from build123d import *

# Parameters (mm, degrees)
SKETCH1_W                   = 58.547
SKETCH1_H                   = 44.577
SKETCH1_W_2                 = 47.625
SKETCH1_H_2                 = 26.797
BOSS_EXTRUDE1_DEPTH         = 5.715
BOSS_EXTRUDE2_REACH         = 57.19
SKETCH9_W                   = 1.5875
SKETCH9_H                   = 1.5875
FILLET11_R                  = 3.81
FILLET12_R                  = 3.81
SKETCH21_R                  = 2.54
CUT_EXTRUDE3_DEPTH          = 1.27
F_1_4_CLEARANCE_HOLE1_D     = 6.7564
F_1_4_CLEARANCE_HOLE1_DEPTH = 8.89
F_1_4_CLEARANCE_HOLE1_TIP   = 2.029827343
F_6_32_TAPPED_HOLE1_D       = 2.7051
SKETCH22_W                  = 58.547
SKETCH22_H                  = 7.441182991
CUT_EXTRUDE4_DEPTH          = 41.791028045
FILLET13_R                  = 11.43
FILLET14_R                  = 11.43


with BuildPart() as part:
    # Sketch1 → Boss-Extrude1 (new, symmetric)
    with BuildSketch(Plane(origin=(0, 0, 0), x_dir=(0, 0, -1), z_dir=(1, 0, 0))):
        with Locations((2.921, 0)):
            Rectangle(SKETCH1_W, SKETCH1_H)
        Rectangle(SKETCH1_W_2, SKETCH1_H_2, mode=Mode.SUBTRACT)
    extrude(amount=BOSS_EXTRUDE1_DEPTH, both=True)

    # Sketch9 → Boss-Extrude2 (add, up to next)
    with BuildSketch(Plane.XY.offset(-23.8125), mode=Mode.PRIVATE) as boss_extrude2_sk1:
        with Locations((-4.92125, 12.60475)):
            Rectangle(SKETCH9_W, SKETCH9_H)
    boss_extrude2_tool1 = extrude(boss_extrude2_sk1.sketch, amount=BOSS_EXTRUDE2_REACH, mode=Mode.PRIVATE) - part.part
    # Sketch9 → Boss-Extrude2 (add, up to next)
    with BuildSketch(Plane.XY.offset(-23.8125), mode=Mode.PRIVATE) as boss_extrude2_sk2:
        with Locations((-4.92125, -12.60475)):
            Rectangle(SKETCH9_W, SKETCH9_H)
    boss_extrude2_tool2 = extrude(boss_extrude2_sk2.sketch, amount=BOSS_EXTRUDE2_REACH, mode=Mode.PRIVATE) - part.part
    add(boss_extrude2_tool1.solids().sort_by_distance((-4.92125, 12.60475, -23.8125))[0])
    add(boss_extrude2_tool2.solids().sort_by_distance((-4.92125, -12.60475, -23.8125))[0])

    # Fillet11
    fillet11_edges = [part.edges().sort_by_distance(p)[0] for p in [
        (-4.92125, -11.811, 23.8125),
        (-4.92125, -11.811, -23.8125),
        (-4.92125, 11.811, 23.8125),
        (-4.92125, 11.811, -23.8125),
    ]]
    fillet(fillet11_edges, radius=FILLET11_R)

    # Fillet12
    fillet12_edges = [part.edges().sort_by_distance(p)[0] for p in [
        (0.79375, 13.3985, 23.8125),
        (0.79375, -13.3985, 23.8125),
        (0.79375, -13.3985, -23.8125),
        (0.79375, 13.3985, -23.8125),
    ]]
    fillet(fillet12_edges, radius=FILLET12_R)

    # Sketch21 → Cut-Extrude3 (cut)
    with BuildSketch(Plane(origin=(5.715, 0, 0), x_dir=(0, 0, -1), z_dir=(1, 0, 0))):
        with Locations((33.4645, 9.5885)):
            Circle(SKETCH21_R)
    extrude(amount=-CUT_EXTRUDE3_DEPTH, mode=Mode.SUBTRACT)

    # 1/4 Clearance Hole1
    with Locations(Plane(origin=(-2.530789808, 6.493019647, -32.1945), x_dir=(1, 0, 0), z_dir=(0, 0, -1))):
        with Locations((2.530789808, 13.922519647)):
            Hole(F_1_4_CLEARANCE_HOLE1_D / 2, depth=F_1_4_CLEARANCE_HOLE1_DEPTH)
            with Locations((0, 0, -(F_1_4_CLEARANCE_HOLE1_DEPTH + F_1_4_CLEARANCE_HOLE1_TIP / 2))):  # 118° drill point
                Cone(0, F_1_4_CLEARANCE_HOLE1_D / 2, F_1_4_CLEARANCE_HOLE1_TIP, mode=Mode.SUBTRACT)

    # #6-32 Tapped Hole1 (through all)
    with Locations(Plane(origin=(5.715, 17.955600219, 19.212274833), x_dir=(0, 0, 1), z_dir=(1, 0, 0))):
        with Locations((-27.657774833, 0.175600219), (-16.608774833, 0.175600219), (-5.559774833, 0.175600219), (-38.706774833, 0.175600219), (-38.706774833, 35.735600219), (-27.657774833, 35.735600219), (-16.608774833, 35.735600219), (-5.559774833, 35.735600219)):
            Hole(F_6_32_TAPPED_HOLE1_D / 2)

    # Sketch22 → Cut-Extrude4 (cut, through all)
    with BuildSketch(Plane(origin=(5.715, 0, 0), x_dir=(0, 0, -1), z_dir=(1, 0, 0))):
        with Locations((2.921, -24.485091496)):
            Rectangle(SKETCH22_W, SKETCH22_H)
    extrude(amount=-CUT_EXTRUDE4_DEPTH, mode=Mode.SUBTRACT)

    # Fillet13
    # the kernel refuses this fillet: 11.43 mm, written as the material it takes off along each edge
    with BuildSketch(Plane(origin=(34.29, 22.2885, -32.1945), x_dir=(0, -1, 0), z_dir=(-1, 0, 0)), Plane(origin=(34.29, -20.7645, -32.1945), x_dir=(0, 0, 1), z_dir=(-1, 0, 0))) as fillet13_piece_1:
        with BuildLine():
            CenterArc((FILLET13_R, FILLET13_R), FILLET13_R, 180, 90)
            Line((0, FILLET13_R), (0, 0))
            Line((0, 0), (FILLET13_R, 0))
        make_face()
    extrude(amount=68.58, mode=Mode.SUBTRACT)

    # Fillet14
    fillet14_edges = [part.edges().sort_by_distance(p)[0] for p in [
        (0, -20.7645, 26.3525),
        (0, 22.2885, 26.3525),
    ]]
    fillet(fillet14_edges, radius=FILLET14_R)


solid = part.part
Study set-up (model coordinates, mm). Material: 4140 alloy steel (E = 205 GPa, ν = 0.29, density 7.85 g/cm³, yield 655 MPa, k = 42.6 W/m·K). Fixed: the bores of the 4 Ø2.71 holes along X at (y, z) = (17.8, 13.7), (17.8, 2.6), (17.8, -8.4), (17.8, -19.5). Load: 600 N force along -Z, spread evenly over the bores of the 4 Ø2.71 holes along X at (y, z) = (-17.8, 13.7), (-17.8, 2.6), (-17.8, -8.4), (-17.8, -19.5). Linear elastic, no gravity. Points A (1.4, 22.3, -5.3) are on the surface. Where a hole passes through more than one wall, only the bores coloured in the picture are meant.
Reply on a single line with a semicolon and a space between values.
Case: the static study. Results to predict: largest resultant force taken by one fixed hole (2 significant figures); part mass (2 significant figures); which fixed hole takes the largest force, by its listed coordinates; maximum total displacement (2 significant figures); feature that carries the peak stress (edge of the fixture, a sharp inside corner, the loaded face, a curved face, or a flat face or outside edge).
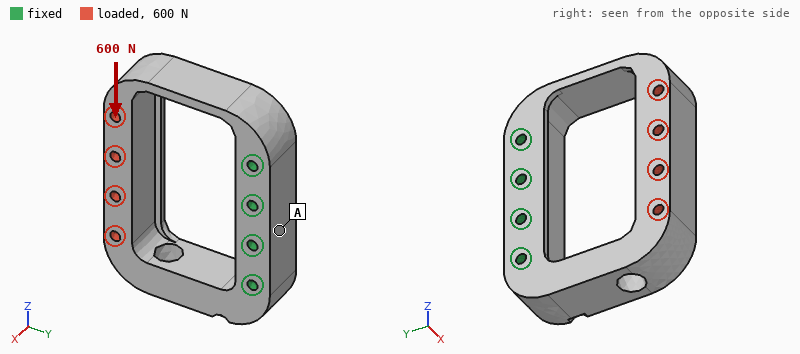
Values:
830 N; 98 g; (17.8, -19.5); 49 µm; a sharp inside corner
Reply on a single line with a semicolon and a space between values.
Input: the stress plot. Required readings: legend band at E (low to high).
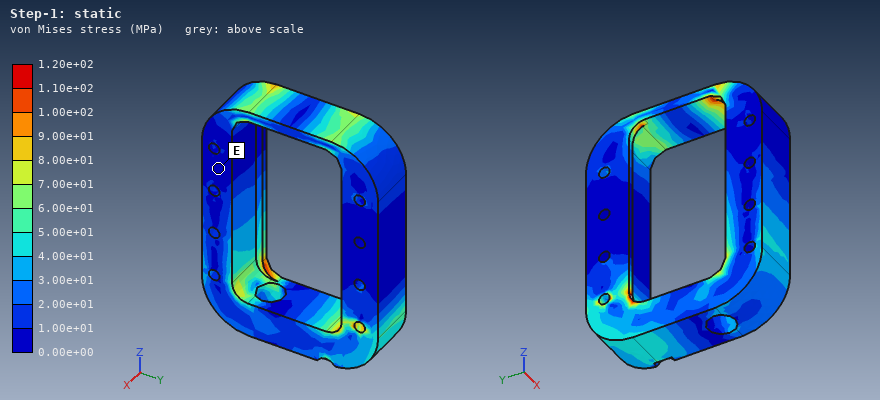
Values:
0.00e+00 to 1.00e+01 MPa
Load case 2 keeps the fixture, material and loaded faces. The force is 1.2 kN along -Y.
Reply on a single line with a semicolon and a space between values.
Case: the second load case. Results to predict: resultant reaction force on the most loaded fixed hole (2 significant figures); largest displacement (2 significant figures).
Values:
840 N; 31 µm
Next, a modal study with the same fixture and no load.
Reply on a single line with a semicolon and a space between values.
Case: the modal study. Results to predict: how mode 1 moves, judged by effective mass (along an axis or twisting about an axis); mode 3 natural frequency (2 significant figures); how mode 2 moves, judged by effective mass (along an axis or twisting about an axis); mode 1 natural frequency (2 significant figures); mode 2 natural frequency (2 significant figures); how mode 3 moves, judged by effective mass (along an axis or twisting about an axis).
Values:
along X; 5500 Hz; along Z; 2600 Hz; 2800 Hz; twisting about Y
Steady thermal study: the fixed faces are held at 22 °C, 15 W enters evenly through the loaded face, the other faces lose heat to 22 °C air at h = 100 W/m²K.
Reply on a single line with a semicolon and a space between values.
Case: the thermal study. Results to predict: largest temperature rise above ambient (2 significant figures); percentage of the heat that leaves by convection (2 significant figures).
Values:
50 K; 79 %
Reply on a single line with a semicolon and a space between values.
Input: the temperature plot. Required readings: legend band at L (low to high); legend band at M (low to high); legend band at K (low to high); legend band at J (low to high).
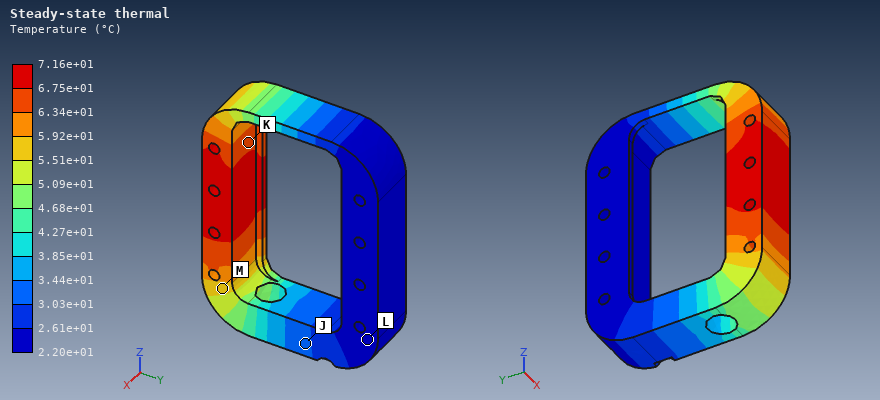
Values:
2.20e+01 to 2.61e+01 °C; 5.51e+01 to 5.92e+01 °C; 6.34e+01 to 6.75e+01 °C; 3.03e+01 to 3.44e+01 °C
